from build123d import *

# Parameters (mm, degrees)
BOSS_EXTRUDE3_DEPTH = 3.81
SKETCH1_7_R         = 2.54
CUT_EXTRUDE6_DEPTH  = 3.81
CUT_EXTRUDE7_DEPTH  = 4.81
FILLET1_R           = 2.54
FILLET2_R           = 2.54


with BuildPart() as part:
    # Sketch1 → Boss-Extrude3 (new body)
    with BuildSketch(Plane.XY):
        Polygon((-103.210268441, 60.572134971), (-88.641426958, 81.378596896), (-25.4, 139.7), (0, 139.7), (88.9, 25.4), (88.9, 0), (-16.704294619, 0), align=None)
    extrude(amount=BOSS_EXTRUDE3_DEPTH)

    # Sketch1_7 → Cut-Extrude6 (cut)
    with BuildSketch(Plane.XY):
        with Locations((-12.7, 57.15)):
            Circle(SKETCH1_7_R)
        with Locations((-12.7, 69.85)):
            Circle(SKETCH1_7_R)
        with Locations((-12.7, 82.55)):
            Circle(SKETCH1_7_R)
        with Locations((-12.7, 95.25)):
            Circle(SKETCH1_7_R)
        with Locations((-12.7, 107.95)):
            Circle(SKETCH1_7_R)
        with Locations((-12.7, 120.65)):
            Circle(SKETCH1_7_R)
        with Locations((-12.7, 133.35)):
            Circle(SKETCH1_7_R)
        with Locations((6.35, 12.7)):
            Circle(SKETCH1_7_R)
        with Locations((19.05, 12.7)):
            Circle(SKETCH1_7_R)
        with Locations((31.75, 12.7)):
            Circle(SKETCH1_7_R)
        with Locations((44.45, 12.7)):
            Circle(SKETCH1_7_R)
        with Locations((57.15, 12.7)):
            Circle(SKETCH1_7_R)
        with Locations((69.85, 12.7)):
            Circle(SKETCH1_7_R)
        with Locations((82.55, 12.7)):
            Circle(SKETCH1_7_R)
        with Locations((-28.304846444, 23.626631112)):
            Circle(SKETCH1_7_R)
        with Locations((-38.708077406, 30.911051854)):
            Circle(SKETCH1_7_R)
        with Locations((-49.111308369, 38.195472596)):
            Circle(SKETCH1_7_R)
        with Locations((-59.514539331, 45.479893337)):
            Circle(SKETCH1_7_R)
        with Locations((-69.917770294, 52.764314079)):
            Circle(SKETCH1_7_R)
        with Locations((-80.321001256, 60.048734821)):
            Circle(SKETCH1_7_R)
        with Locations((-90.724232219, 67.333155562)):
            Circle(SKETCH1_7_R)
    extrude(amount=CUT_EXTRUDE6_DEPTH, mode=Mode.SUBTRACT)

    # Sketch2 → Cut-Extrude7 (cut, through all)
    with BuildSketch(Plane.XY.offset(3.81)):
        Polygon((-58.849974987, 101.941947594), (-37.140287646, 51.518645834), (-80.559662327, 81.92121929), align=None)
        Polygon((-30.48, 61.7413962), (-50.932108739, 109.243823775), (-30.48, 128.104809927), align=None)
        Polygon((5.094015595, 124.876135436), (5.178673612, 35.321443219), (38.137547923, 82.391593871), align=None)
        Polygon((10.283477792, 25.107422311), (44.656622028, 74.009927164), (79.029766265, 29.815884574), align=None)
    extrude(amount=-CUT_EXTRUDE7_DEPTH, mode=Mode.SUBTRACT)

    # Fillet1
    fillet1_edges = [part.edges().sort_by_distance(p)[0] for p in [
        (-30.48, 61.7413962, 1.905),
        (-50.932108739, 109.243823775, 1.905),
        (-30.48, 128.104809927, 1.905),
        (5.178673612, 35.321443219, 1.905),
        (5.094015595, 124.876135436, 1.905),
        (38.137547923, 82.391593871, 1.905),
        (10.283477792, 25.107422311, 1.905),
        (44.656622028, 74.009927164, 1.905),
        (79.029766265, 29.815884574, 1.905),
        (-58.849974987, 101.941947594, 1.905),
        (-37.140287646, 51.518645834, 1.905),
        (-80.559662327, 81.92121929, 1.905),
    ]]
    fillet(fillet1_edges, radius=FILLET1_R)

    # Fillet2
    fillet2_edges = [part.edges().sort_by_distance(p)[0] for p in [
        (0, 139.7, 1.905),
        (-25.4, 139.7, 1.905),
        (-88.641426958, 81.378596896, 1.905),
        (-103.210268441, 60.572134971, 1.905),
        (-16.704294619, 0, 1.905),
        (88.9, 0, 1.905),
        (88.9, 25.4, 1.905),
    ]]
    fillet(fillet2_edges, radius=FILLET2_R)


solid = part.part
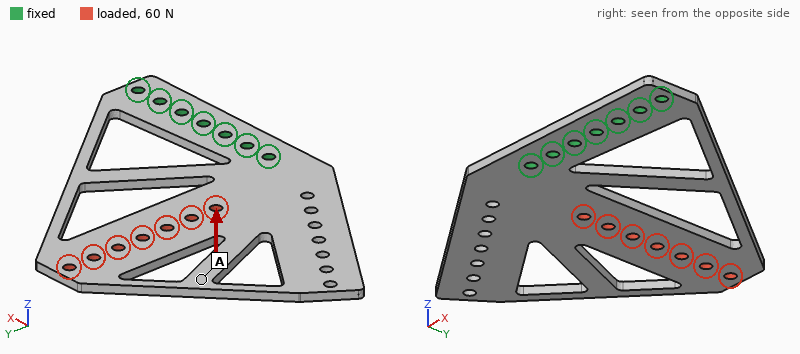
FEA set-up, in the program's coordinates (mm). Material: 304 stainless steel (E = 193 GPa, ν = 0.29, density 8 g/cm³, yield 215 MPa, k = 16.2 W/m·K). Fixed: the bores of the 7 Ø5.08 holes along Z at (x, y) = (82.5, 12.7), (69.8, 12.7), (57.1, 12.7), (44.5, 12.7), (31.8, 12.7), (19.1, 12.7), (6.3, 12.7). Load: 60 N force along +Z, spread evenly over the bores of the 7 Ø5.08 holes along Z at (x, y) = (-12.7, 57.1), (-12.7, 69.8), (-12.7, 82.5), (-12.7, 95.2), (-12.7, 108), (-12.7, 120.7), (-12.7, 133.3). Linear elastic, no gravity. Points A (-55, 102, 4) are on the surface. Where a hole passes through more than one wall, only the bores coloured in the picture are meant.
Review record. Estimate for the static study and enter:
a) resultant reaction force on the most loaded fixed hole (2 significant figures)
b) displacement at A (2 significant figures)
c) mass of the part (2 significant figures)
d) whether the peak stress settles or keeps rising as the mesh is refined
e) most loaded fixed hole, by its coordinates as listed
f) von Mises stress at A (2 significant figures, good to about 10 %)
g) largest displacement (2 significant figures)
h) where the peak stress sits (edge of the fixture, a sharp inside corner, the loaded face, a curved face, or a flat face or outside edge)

95 N
0.35 mm
350 g
keeps rising
(6.3, 12.7)
6.2 MPa
0.52 mm
edge of the fixture
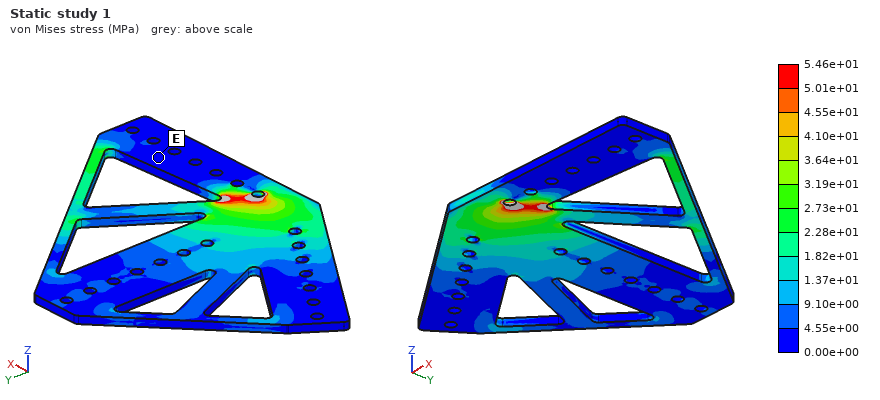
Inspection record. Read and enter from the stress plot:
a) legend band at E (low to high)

0.00e+00 to 4.55e+00 MPa
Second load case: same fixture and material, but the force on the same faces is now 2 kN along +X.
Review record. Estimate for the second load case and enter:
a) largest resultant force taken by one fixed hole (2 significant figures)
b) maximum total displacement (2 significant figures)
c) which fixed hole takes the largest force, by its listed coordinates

3.6 kN
0.12 mm
(6.3, 12.7)
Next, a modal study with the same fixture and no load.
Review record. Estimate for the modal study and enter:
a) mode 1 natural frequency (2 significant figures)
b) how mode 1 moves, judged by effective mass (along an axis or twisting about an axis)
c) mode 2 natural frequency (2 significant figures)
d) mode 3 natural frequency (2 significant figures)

170 Hz
along Z
330 Hz
930 Hz
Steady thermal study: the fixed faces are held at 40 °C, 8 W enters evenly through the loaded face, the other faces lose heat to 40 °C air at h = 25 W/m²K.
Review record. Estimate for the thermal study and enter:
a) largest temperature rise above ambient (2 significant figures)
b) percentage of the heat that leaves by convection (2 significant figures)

40 K
94 %
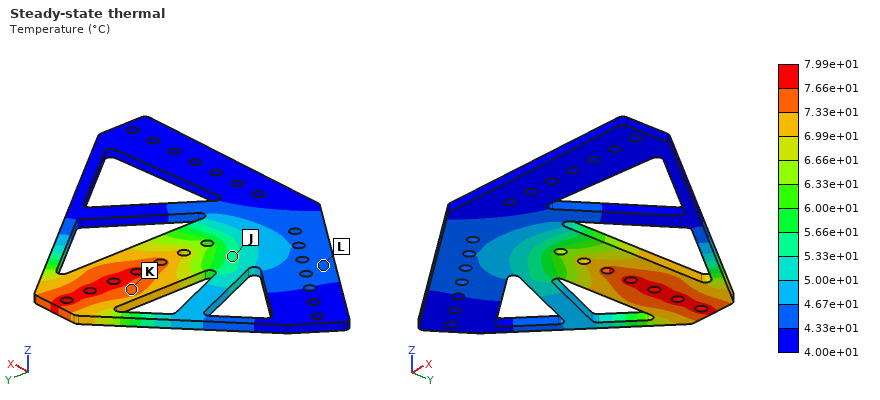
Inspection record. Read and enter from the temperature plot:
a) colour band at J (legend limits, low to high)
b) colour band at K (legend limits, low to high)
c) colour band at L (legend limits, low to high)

5.33e+01 to 5.66e+01 °C
7.33e+01 to 7.66e+01 °C
4.33e+01 to 4.67e+01 °C
